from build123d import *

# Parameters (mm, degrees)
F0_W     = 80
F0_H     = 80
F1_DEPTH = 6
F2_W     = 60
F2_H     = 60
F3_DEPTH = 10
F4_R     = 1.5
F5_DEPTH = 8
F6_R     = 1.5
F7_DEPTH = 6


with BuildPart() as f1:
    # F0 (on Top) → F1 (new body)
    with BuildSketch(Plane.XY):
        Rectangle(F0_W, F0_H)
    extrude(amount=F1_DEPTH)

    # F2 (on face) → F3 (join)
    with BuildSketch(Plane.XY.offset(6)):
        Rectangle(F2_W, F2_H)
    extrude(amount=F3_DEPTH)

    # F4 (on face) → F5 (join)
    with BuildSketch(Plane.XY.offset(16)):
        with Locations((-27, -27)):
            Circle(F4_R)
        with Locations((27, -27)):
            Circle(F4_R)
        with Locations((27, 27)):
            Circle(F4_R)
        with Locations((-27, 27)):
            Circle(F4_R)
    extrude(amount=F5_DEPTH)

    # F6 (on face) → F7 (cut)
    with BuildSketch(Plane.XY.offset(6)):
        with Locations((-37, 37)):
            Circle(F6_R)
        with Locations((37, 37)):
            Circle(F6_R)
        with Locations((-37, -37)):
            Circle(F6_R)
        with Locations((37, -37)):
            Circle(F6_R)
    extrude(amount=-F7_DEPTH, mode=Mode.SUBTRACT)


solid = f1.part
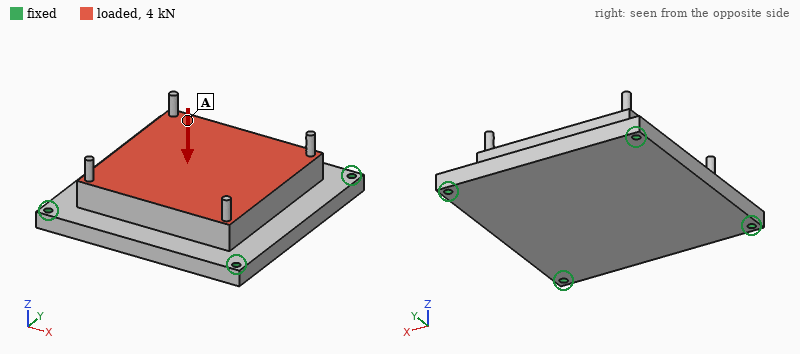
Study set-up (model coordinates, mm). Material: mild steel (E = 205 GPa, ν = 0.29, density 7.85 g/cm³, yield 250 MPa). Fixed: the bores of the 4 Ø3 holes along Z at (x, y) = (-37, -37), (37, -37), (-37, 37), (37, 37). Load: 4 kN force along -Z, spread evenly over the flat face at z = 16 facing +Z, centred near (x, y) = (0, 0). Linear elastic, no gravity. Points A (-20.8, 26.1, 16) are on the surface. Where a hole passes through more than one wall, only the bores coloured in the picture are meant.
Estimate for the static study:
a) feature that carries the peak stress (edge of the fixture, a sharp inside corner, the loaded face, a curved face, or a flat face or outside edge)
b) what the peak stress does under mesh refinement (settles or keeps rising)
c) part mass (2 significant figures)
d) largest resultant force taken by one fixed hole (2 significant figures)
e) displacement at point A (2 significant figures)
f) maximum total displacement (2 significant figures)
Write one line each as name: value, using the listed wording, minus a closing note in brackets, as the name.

feature that carries the peak stress: edge of the fixture
what the peak stress does under mesh refinement: keeps rising
part mass: 580 g
largest resultant force taken by one fixed hole: 1.2 kN
displacement at point A: 10 µm
maximum total displacement: 13 µm
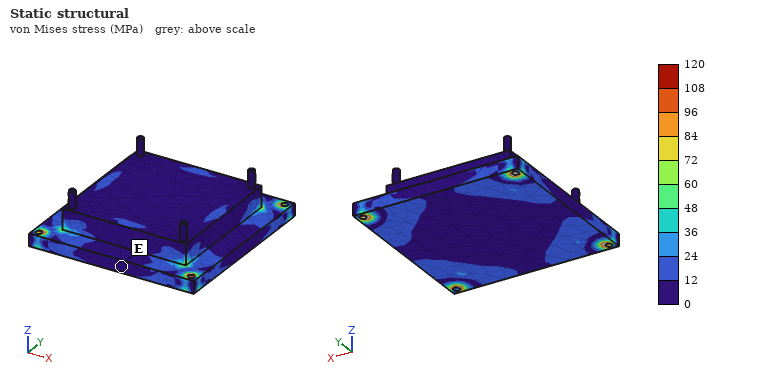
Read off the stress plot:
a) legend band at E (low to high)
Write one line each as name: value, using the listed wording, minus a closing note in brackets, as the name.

legend band at E: 0 to 12 MPa
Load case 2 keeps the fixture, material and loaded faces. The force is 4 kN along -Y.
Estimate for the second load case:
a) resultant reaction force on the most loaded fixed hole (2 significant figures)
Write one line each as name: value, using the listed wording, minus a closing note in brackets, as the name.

resultant reaction force on the most loaded fixed hole: 1.2 kN
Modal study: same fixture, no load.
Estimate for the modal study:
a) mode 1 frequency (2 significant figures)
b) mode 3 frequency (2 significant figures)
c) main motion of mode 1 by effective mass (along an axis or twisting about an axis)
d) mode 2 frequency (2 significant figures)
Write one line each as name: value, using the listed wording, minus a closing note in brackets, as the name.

mode 1 frequency: 4000 Hz
mode 3 frequency: 7000 Hz
main motion of mode 1 by effective mass: along Z
mode 2 frequency: 7000 Hz
